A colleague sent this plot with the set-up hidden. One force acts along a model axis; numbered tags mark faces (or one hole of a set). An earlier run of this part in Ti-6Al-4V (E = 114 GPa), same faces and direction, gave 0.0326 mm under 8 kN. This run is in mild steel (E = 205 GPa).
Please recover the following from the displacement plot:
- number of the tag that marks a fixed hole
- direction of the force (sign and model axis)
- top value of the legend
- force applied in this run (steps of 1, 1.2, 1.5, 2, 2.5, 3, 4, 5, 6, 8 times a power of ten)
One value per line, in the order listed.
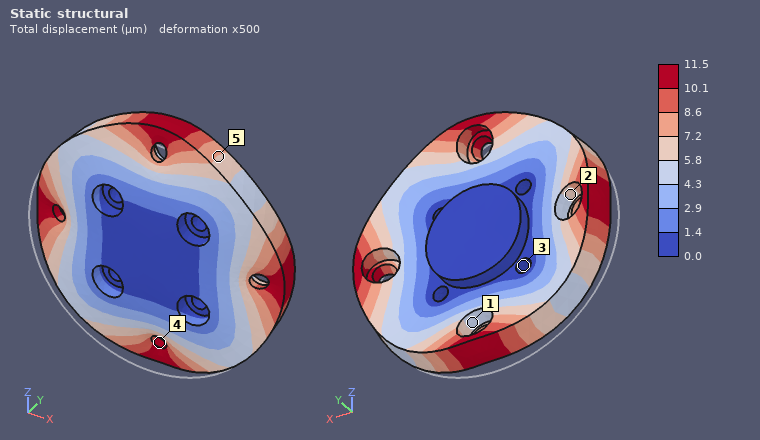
3
+Y
11.5 µm
5 kN
